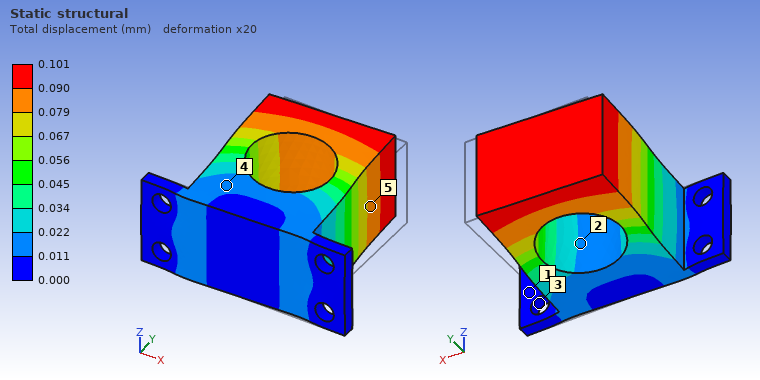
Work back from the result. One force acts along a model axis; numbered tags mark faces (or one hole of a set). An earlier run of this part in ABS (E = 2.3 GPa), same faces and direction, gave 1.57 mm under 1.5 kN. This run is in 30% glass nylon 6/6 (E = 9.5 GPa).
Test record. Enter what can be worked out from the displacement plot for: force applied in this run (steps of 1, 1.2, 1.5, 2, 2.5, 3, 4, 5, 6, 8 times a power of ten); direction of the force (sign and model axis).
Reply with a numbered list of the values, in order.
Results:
1. 400 N
2. -X
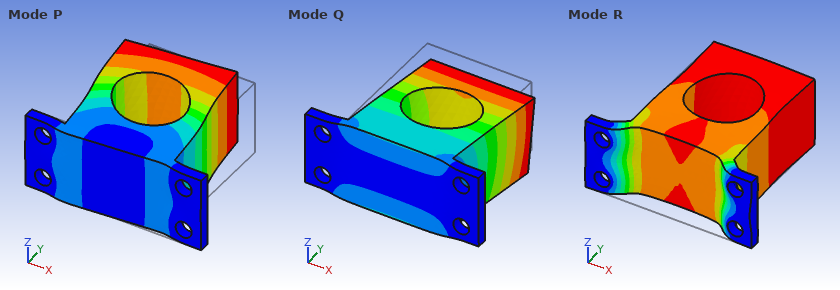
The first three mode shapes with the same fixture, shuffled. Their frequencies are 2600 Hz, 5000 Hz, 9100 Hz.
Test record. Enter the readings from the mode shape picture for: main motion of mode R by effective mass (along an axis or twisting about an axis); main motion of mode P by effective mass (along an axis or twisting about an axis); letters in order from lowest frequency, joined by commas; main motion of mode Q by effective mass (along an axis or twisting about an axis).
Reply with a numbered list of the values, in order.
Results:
1. along Y
2. along X
3. Q, P, R
4. along Z
